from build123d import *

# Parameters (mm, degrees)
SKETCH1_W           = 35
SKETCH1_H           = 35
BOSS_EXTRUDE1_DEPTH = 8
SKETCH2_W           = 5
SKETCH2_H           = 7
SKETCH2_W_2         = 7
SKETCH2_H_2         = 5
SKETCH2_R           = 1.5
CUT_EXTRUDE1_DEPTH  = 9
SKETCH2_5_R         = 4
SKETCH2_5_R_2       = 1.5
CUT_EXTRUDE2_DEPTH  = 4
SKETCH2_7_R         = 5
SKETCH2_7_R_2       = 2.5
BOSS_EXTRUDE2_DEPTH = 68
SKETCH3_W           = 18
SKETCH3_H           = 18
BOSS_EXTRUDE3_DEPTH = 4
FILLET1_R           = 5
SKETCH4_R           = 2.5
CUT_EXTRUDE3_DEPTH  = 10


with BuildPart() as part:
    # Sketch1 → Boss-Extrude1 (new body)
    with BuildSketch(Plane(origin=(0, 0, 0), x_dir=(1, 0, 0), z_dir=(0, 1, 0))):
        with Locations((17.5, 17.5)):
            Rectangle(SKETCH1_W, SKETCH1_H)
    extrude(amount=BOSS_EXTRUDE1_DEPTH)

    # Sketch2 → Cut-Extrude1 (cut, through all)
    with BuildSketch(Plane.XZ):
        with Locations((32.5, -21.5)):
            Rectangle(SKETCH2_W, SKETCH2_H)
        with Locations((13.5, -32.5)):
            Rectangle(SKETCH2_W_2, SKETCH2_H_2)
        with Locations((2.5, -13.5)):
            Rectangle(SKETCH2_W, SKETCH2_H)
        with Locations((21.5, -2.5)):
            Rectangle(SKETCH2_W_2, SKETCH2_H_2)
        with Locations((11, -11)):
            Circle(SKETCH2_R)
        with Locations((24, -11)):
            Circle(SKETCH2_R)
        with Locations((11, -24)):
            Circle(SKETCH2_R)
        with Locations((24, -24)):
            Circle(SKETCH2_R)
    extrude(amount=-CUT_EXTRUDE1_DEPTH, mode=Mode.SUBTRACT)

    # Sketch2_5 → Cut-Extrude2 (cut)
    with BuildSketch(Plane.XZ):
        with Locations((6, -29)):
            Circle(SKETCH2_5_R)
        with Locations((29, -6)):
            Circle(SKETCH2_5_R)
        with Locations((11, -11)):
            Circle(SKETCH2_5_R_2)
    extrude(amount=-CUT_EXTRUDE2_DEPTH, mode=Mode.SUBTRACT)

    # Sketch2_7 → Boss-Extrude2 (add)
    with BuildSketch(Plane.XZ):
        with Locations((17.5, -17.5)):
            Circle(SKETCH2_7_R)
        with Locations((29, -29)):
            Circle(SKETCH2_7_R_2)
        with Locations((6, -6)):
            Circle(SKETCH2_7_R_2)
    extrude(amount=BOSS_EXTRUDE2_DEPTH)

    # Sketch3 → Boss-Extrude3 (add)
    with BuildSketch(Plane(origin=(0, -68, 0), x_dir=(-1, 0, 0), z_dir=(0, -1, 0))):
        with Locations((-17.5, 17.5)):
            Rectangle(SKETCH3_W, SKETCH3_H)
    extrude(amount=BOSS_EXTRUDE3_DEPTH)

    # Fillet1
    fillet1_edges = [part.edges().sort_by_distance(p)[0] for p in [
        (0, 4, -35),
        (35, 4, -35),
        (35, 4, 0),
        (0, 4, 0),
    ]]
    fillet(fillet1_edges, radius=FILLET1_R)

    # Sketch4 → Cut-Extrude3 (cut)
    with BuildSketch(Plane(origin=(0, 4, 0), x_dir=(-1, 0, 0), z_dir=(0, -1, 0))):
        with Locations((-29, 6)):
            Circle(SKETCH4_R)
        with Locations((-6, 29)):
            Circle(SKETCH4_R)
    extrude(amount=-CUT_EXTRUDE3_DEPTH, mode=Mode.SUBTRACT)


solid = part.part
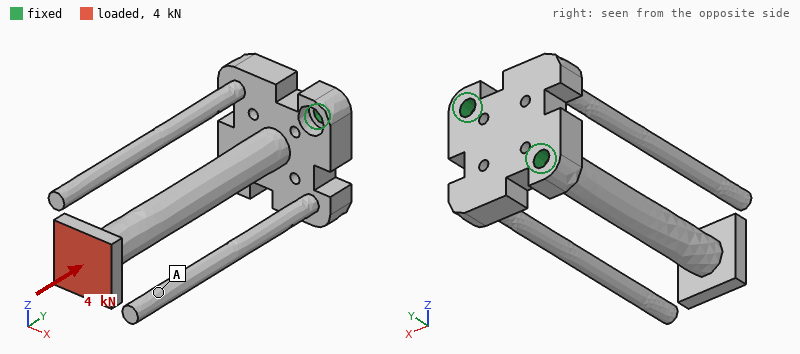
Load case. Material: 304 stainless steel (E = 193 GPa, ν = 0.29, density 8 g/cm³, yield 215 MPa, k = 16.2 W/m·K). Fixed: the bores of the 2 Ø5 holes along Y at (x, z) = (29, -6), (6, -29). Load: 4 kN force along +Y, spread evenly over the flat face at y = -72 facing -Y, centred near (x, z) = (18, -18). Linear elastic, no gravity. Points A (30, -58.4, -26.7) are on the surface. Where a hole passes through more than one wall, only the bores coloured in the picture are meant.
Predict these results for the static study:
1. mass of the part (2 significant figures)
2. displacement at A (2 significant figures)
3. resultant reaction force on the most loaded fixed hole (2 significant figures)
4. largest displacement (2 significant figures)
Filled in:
140 g
15 µm
2.4 kN
35 µm
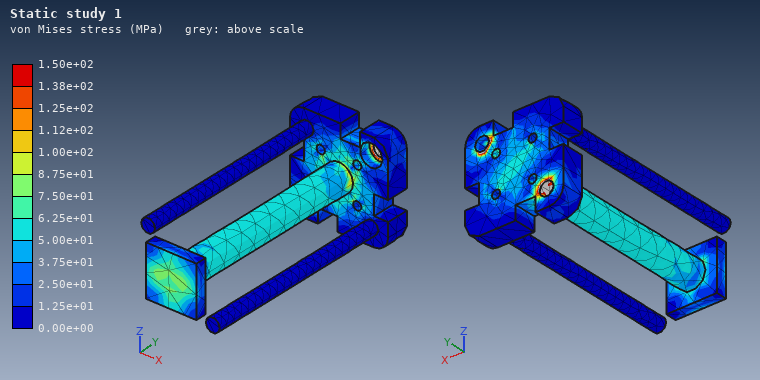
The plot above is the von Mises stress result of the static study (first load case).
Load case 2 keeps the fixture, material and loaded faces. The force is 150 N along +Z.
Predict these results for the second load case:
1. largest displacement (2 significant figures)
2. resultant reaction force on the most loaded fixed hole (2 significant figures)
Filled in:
0.27 mm
310 N
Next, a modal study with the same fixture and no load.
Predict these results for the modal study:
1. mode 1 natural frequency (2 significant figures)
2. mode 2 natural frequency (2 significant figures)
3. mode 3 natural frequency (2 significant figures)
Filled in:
670 Hz
700 Hz
710 Hz
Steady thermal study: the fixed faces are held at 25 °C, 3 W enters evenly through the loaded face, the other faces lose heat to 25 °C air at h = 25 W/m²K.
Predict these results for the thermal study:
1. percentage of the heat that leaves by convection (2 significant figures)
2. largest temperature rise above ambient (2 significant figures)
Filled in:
83 %
68 K
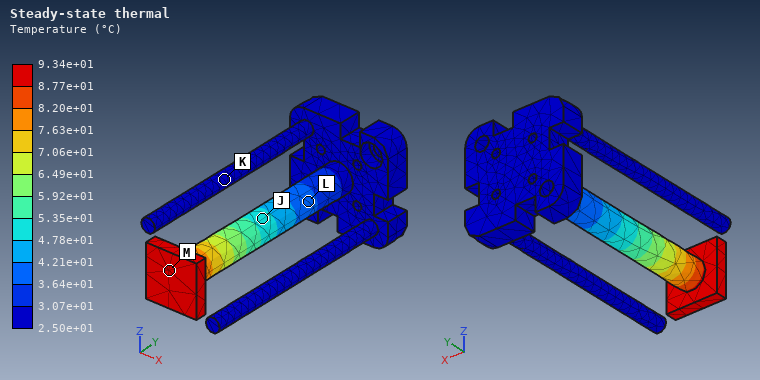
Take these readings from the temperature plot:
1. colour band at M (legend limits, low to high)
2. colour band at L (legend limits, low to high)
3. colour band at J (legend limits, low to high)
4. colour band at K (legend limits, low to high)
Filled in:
8.77e+01 to 9.34e+01 °C
3.64e+01 to 4.21e+01 °C
4.78e+01 to 5.35e+01 °C
2.50e+01 to 3.07e+01 °C
